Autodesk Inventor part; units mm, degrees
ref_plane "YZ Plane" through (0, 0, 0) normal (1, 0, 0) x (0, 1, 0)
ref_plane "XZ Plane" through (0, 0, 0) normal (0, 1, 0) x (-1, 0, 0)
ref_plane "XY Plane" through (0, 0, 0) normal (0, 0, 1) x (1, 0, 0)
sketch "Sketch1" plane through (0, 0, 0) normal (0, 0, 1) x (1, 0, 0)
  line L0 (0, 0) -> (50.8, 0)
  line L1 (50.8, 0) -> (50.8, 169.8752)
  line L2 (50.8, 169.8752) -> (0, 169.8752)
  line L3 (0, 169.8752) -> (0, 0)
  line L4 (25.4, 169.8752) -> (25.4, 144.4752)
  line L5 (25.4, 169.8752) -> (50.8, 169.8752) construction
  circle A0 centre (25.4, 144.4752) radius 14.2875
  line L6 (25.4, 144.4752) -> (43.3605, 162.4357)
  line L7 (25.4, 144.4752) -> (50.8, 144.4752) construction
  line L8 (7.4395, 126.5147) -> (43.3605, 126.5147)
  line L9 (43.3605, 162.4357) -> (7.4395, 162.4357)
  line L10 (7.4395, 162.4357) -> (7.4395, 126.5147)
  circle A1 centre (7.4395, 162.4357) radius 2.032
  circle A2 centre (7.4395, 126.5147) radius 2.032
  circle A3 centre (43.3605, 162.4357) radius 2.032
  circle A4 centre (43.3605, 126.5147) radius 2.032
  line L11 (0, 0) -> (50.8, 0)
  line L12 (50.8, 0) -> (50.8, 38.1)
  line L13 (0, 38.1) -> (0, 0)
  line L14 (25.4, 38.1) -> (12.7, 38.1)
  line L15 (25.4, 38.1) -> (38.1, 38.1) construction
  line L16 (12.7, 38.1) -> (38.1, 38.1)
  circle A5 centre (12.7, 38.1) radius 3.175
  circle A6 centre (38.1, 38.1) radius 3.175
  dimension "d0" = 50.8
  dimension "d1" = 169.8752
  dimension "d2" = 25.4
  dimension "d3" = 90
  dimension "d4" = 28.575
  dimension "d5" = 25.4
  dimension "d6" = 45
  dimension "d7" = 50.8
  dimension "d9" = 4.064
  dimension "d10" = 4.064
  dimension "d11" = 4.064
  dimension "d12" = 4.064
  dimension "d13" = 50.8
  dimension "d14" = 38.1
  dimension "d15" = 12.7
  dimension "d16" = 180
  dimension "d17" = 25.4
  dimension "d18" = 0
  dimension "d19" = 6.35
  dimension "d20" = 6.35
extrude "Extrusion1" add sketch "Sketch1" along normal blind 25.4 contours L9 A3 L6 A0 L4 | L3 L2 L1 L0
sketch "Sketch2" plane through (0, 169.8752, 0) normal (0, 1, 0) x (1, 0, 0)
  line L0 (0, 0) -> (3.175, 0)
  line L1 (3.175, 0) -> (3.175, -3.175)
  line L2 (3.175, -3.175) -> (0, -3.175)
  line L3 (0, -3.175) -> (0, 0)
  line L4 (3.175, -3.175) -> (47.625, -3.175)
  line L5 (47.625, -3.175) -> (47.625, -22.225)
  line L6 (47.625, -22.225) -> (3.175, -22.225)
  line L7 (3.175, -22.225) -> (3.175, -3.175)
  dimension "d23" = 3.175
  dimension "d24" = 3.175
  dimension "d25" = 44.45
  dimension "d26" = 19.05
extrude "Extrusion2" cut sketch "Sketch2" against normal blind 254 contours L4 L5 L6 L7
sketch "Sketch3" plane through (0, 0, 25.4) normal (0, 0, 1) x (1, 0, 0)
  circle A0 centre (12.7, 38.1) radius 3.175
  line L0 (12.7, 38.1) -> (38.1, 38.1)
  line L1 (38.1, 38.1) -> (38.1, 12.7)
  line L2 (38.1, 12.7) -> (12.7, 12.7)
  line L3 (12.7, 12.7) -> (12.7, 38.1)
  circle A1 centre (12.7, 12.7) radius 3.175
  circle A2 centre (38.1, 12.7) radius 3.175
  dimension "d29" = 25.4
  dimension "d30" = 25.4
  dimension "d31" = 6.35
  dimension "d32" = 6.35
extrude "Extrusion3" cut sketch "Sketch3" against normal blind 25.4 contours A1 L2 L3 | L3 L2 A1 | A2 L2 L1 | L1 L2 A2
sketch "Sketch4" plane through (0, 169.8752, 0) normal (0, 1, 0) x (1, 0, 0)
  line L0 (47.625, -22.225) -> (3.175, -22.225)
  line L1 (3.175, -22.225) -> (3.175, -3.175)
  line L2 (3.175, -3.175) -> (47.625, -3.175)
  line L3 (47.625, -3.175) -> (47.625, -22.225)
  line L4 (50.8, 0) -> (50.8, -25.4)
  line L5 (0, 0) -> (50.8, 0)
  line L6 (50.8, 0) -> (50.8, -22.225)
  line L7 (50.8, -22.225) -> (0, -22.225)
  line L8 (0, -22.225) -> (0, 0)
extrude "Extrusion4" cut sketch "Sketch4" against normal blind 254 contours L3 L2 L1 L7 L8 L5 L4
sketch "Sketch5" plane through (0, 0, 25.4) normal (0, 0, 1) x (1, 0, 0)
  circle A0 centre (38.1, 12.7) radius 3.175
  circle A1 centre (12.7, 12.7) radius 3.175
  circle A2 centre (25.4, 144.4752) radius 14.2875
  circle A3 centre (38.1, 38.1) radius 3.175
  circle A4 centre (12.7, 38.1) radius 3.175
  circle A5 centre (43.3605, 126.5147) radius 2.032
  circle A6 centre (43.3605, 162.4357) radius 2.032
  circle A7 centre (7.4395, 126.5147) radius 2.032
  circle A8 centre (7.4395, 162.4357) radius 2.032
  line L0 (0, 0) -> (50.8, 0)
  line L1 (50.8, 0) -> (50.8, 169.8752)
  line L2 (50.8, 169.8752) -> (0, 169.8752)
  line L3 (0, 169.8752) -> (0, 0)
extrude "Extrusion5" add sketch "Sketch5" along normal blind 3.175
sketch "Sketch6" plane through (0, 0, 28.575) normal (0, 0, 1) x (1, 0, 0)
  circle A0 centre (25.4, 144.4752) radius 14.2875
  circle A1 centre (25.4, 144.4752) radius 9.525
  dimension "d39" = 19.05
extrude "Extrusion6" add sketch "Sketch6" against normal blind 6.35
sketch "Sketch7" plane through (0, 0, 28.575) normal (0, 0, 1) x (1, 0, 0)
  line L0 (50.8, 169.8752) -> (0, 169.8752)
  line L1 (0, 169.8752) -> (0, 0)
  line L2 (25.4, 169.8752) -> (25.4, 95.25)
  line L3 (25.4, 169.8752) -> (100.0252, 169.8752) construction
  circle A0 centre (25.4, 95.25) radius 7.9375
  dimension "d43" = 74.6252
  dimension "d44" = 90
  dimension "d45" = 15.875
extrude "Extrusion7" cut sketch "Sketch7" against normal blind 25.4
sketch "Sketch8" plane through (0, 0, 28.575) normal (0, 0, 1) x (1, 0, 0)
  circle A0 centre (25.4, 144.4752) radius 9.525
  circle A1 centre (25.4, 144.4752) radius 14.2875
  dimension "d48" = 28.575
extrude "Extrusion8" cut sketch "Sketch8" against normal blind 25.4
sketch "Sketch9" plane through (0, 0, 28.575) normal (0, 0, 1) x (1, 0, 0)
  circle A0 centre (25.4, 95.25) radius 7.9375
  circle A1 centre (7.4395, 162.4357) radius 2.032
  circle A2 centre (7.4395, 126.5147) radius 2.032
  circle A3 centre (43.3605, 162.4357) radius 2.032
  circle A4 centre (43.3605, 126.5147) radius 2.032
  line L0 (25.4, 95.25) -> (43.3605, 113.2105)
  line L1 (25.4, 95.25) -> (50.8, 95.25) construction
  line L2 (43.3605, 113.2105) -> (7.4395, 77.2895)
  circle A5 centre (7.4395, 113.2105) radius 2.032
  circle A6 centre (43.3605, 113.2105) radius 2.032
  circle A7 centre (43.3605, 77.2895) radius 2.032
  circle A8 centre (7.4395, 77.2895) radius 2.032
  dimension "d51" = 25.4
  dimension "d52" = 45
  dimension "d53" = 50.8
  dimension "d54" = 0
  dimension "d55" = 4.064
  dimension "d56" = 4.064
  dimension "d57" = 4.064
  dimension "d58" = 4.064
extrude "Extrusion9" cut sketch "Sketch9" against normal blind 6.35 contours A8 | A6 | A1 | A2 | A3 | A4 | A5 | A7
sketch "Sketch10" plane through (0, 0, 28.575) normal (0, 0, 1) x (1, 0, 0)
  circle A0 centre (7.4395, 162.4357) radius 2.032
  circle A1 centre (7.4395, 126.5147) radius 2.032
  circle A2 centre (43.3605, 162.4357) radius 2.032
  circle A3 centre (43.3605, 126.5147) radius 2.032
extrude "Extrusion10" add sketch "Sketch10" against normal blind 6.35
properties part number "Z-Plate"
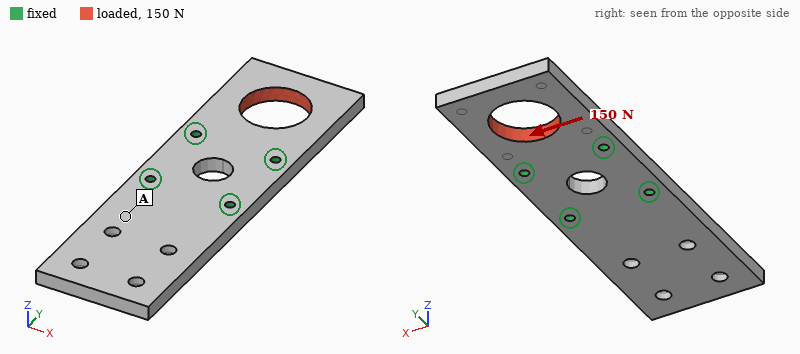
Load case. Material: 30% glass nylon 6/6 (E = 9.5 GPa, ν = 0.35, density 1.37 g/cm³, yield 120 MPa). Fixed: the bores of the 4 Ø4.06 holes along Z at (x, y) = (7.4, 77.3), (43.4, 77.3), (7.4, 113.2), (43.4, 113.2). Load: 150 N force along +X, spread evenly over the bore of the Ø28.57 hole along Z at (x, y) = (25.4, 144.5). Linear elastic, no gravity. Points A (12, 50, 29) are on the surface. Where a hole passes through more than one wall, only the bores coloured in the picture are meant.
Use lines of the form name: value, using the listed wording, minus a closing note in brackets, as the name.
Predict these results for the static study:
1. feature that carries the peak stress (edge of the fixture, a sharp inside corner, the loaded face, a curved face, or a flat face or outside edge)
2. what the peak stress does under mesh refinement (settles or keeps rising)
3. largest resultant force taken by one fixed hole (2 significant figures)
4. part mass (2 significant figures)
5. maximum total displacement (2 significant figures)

feature that carries the peak stress: edge of the fixture
what the peak stress does under mesh refinement: keeps rising
largest resultant force taken by one fixed hole: 130 N
part mass: 66 g
maximum total displacement: 26 µm
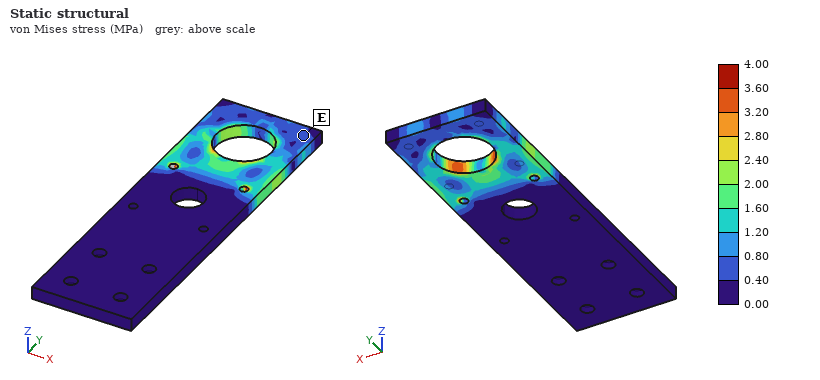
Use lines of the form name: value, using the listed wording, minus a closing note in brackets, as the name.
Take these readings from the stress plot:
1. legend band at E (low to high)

legend band at E: 0.40 to 0.80 MPa
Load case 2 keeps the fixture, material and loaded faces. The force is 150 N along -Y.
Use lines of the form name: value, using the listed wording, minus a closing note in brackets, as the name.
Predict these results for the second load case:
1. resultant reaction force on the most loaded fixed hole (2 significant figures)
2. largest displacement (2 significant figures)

resultant reaction force on the most loaded fixed hole: 67 N
largest displacement: 5.3 µm
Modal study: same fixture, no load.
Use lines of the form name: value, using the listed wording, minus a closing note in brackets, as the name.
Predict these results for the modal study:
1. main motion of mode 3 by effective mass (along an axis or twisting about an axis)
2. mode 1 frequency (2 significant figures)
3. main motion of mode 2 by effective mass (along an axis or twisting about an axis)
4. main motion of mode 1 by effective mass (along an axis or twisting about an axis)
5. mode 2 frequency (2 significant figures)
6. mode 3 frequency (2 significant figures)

main motion of mode 3 by effective mass: twisting about Y
mode 1 frequency: 440 Hz
main motion of mode 2 by effective mass: along Z
main motion of mode 1 by effective mass: along Z
mode 2 frequency: 770 Hz
mode 3 frequency: 1500 Hz
